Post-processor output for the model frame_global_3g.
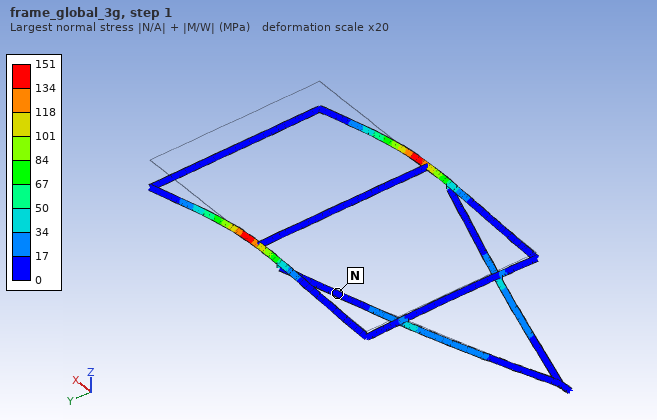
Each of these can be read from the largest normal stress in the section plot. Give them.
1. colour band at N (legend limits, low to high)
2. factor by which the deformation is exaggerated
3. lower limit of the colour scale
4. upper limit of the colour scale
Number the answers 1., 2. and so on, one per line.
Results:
1. 0 to 17 MPa
2. 20
3. 0 MPa
4. 151 MPa
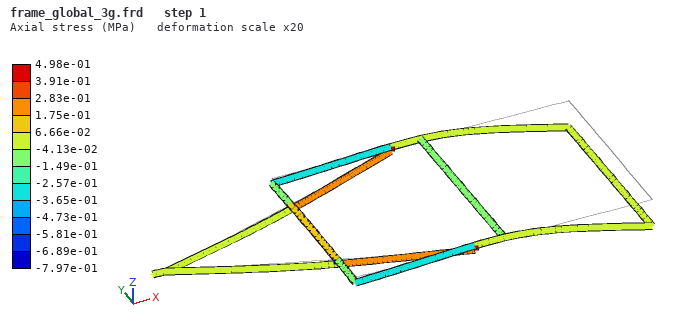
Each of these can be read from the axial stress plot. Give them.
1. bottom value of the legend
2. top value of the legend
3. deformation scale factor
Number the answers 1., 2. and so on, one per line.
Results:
1. -7.97e-01 MPa
2. 4.98e-01 MPa
3. 20
